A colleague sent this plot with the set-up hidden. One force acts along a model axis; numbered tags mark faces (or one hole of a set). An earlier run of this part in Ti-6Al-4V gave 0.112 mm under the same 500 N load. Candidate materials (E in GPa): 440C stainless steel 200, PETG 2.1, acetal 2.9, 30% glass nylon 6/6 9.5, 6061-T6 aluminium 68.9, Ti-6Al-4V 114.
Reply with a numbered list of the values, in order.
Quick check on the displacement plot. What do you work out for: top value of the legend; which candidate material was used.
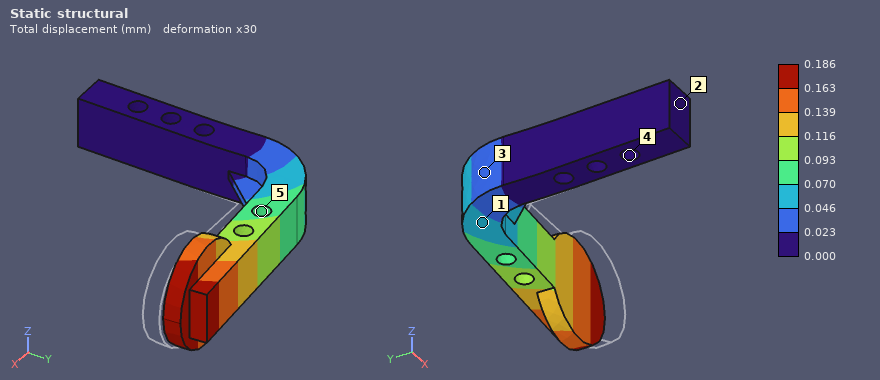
1. 0.186 mm
2. 6061-T6 aluminium
